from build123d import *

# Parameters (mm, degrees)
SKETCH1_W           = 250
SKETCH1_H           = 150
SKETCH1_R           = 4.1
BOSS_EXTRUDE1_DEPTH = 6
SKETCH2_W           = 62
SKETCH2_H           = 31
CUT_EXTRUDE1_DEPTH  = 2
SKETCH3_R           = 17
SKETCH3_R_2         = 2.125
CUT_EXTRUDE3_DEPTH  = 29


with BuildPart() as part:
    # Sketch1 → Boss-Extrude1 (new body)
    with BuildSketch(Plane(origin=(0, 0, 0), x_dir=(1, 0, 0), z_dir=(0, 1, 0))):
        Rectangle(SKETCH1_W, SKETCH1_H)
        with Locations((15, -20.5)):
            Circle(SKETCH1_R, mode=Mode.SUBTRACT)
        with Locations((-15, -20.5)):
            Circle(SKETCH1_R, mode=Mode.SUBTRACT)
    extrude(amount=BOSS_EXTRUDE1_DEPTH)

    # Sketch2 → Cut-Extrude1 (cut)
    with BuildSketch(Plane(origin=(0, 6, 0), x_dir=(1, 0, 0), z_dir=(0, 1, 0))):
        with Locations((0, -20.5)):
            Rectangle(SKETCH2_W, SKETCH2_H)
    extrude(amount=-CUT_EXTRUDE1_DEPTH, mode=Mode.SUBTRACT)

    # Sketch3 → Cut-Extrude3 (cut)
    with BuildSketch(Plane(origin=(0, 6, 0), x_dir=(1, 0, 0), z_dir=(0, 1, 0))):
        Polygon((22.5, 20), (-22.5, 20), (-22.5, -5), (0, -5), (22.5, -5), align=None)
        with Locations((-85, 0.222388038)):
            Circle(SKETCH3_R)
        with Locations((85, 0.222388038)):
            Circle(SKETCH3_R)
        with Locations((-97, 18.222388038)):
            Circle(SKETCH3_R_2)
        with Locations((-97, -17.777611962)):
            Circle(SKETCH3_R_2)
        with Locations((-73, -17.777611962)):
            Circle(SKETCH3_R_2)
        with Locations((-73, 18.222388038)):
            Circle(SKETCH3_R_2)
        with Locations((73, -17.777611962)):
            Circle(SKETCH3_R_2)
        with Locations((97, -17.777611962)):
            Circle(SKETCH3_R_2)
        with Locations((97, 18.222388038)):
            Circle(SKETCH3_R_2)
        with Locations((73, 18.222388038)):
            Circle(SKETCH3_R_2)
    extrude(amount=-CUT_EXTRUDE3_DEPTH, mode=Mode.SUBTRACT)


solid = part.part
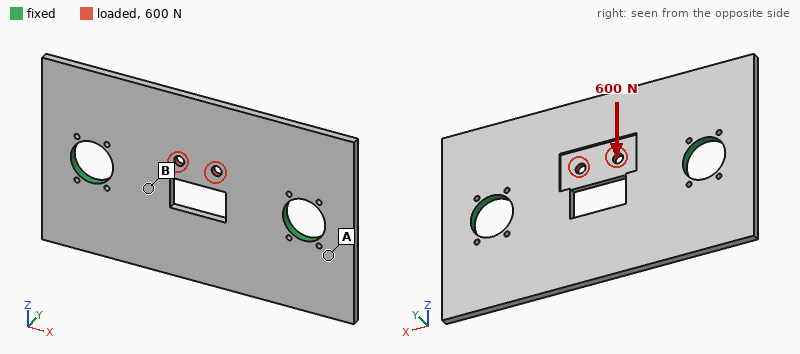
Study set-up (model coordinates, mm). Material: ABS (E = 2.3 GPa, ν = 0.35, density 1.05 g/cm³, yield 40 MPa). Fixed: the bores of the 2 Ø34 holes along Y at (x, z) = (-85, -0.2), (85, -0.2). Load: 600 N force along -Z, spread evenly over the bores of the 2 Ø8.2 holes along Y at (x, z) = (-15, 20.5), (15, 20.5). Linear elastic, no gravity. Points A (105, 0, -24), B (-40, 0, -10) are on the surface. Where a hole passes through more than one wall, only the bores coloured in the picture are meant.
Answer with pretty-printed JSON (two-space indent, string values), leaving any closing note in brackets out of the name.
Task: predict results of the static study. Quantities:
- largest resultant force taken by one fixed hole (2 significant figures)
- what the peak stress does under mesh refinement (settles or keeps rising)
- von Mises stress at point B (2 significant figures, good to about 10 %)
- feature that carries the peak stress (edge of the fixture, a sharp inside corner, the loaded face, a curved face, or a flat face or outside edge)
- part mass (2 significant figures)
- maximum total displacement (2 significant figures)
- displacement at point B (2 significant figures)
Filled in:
{
  "largest resultant force taken by one fixed hole": "310 N",
  "what the peak stress does under mesh refinement": "keeps rising",
  "von Mises stress at point B": "1.1 MPa",
  "feature that carries the peak stress": "a sharp inside corner",
  "part mass": "210 g",
  "maximum total displacement": "0.15 mm",
  "displacement at point B": "0.028 mm"
}
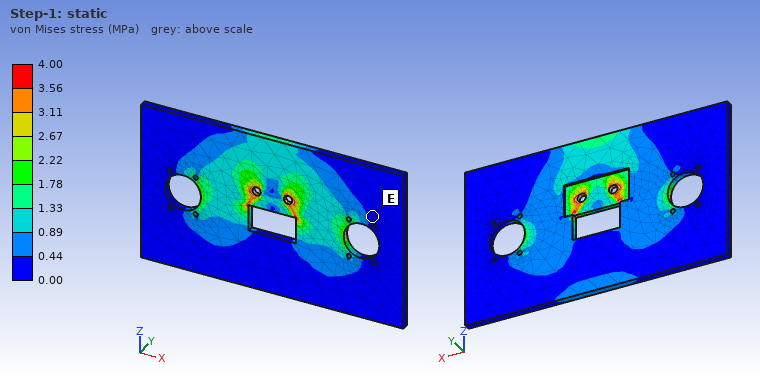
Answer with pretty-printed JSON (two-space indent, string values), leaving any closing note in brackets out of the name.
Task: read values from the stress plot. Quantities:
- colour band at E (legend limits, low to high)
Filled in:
{
  "colour band at E": "0.00 to 0.44 MPa"
}
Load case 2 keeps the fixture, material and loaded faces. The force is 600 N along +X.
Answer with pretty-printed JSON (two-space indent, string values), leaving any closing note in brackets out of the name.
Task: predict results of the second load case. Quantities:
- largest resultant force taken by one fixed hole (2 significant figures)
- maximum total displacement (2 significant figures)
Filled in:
{
  "largest resultant force taken by one fixed hole": "300 N",
  "maximum total displacement": "56 µm"
}
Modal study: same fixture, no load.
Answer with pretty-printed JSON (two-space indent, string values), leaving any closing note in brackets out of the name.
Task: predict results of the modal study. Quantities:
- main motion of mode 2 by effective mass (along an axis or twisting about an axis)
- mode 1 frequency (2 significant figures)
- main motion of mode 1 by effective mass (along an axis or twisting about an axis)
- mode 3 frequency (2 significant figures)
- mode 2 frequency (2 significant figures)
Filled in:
{
  "main motion of mode 2 by effective mass": "along Y",
  "mode 1 frequency": "250 Hz",
  "main motion of mode 1 by effective mass": "twisting about X",
  "mode 3 frequency": "400 Hz",
  "mode 2 frequency": "270 Hz"
}
